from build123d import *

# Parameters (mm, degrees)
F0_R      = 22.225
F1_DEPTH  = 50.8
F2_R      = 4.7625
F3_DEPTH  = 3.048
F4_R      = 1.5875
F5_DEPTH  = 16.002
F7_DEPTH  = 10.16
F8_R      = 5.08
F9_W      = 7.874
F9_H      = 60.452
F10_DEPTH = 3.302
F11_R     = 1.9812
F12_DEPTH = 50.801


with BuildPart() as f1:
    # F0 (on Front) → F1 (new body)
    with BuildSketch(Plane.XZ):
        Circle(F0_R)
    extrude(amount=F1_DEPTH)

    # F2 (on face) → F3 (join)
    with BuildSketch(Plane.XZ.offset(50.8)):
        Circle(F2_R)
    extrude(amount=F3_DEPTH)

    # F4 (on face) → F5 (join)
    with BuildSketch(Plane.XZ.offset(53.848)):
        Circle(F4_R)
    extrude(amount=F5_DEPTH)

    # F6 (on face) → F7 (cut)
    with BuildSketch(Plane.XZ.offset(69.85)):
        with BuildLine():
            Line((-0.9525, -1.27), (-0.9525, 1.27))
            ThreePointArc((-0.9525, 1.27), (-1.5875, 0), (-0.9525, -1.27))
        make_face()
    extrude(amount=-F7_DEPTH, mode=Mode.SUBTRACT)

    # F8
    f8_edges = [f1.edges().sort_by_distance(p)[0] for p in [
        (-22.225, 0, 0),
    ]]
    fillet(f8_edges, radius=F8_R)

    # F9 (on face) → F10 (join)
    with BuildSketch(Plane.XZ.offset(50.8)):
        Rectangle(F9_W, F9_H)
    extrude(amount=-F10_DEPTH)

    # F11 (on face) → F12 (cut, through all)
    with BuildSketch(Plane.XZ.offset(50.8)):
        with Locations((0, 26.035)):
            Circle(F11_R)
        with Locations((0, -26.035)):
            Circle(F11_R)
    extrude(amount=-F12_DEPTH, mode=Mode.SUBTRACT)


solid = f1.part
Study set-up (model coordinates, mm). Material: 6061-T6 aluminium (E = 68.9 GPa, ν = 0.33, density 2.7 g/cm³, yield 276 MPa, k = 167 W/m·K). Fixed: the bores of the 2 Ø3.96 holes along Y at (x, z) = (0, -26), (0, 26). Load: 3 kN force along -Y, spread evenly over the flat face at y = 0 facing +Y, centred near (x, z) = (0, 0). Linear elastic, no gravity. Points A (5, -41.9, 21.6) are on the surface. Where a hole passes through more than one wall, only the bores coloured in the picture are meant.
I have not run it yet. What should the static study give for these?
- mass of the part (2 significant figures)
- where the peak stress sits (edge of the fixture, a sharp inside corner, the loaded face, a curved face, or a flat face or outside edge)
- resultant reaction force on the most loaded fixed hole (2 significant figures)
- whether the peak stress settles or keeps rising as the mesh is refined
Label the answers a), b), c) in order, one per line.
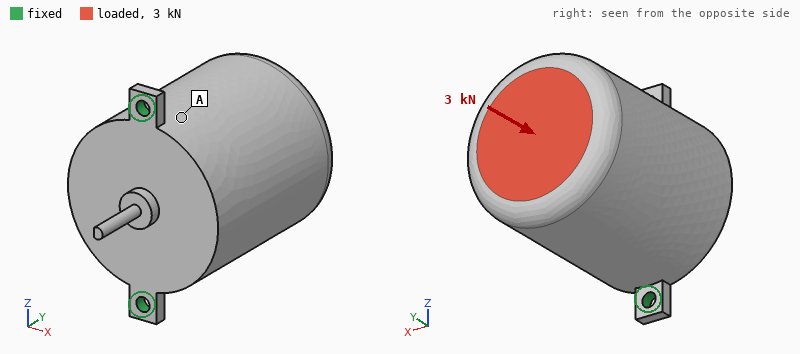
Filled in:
a) 210 g
b) edge of the fixture
c) 1.7 kN
d) keeps rising
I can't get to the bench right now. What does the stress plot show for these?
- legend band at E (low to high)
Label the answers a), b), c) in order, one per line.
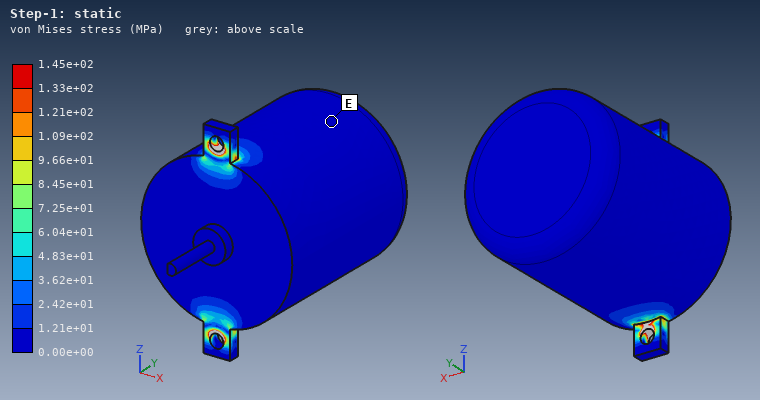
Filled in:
a) 0.00e+00 to 1.21e+01 MPa
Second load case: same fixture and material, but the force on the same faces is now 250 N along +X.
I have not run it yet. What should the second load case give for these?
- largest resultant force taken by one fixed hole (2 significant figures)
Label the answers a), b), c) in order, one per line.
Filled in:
a) 130 N
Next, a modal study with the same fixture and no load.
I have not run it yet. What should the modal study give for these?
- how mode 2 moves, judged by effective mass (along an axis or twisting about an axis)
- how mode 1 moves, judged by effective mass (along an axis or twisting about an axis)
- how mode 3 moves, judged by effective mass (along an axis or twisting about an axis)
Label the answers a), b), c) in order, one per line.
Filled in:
a) along Z
b) along X
c) along Y
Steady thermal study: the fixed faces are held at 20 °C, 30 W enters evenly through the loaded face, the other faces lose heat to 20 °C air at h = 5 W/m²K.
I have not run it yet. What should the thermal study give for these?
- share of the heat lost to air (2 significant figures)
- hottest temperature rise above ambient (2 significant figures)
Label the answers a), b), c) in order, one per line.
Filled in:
a) 3.1 %
b) 25 K
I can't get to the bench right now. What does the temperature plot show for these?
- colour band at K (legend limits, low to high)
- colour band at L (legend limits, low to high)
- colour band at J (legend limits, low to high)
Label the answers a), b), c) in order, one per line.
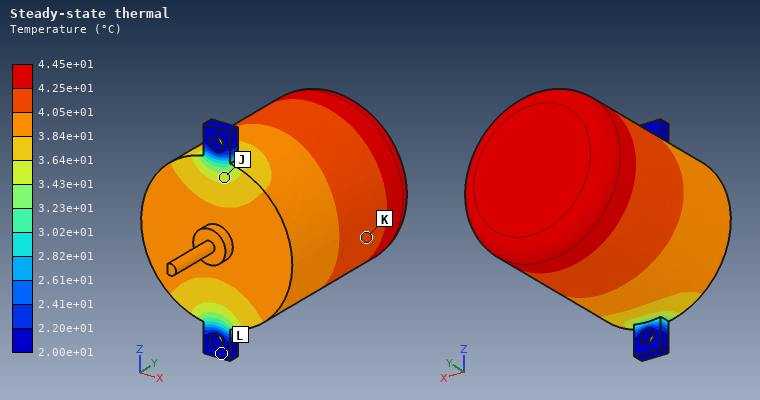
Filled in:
a) 4.05e+01 to 4.25e+01 °C
b) 2.00e+01 to 2.20e+01 °C
c) 3.43e+01 to 3.64e+01 °C
